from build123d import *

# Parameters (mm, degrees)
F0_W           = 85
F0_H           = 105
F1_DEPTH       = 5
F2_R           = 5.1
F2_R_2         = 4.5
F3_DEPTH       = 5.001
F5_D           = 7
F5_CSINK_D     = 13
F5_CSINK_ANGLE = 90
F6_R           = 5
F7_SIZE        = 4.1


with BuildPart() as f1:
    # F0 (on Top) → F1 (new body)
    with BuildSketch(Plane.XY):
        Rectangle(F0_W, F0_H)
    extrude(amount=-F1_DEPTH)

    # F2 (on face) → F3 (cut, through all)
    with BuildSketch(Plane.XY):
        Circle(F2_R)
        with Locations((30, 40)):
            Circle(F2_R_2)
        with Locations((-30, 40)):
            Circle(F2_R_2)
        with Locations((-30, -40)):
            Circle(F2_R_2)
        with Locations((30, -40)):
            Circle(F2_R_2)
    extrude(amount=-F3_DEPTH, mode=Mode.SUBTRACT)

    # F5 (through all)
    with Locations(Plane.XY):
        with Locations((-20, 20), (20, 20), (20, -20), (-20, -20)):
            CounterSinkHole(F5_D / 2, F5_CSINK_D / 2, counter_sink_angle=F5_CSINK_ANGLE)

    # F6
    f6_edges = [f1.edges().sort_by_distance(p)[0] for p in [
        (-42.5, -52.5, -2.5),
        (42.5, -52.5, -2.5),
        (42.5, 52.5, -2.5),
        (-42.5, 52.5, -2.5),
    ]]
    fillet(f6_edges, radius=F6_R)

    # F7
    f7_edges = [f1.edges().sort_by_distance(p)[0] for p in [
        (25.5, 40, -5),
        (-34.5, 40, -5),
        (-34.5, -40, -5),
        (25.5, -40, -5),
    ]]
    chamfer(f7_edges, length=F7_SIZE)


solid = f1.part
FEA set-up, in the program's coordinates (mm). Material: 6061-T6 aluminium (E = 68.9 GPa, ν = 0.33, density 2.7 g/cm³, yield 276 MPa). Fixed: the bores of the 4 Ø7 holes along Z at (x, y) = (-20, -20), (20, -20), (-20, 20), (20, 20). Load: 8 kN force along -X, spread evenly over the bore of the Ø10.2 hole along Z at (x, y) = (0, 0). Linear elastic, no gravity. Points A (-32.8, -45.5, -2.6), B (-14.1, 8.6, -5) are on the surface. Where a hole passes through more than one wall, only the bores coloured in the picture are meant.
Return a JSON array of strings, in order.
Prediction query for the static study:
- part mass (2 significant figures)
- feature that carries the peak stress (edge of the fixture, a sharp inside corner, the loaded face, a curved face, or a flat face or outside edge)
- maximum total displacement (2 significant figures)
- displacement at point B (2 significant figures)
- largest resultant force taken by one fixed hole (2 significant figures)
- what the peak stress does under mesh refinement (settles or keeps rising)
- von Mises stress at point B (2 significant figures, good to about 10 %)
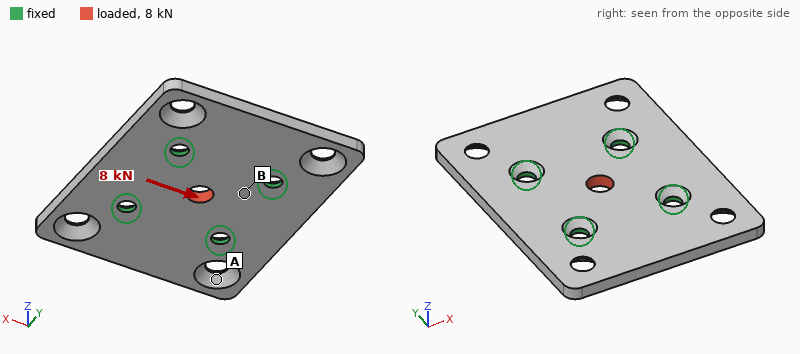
["110 g", "edge of the fixture", "14 µm", "7.0 µm", "2.1 kN", "keeps rising", "30 MPa"]
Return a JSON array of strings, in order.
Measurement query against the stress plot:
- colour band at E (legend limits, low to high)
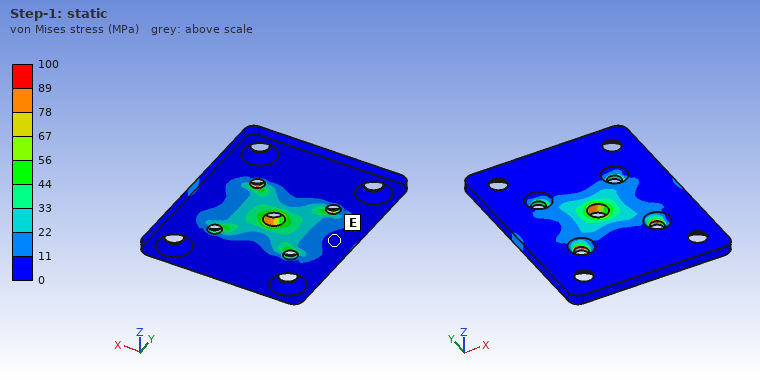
["0 to 11 MPa"]
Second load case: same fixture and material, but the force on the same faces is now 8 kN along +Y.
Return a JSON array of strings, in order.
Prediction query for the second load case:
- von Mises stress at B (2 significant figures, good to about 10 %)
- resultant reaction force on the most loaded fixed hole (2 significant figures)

["26 MPa", "2.1 kN"]
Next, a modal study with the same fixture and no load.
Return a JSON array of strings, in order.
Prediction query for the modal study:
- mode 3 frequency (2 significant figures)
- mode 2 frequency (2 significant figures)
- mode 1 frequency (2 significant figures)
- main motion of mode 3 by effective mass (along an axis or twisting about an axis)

["4100 Hz", "3100 Hz", "3000 Hz", "twisting about Y"]
